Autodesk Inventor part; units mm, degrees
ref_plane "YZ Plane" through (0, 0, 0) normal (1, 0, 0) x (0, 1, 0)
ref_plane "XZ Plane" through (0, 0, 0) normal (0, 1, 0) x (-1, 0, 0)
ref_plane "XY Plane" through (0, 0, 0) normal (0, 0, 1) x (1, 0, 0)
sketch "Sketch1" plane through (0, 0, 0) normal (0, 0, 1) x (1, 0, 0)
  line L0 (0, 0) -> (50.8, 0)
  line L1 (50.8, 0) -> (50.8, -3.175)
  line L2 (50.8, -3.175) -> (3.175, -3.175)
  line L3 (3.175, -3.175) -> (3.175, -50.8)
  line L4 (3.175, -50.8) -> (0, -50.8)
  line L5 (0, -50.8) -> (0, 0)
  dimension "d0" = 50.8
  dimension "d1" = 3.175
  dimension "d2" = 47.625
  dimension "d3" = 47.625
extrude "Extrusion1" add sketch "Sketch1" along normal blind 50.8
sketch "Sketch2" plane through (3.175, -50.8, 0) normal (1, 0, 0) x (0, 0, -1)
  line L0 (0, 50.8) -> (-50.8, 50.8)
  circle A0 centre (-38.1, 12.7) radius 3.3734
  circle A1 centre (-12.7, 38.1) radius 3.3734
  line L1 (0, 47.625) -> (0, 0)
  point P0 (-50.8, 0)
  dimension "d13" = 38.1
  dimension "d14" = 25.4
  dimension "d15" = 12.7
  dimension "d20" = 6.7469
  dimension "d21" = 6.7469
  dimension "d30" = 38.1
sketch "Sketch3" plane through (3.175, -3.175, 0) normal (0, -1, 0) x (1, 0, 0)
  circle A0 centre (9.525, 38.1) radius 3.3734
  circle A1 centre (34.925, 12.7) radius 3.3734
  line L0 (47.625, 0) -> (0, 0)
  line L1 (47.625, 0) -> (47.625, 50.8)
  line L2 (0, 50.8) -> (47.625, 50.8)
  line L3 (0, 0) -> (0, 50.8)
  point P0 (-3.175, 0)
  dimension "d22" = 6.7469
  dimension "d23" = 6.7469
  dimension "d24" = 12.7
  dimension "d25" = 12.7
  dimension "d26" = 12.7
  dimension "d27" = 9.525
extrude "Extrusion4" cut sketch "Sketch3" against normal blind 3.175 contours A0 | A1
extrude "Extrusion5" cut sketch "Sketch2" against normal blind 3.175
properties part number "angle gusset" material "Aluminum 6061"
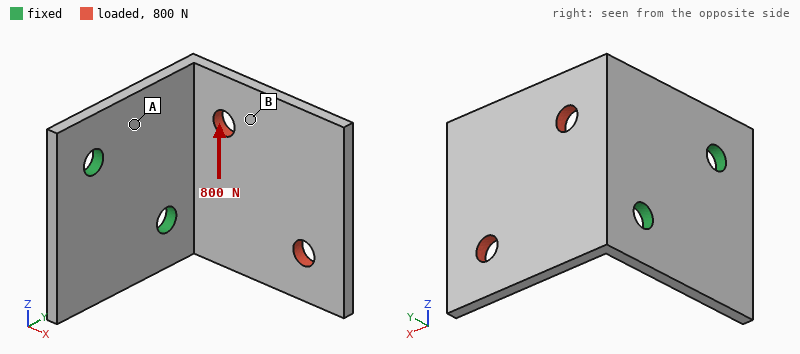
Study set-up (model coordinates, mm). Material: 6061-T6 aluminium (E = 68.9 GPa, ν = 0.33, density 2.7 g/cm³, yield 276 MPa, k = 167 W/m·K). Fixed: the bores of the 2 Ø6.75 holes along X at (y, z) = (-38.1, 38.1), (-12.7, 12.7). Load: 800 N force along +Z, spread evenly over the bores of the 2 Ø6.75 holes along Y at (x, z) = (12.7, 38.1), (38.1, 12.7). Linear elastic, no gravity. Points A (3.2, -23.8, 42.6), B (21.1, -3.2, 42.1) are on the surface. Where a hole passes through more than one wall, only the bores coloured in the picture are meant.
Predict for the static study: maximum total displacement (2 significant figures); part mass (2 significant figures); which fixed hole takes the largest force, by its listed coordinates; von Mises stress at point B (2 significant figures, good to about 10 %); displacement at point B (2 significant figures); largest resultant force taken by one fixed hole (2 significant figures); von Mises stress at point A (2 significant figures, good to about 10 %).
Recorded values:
0.80 mm
42 g
(-12.7, 12.7)
23 MPa
0.42 mm
860 N
63 MPa
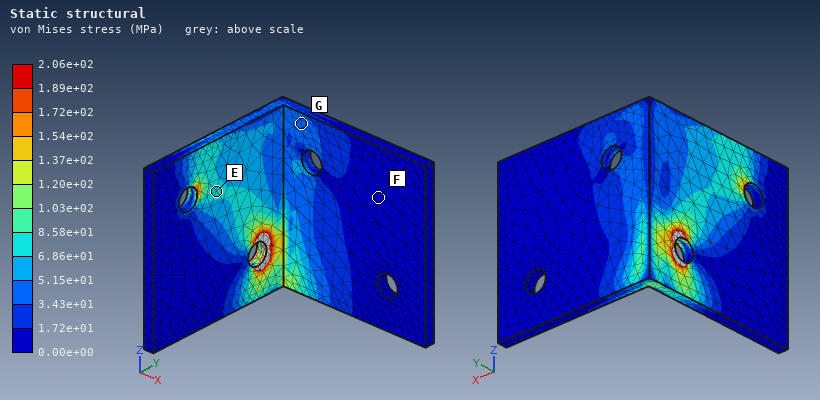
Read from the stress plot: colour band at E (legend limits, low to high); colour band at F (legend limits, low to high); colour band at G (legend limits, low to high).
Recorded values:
6.86e+01 to 8.58e+01 MPa
0.00e+00 to 1.72e+01 MPa
3.43e+01 to 5.15e+01 MPa
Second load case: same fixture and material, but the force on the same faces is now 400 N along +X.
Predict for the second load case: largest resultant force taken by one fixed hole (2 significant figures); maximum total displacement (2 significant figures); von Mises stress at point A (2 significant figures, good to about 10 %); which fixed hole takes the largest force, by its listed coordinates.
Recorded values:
380 N
0.29 mm
22 MPa
(-12.7, 12.7)
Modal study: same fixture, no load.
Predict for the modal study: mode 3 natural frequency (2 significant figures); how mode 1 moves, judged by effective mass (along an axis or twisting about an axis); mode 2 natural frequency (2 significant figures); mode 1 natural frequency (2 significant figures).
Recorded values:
2300 Hz
along Y
1300 Hz
770 Hz
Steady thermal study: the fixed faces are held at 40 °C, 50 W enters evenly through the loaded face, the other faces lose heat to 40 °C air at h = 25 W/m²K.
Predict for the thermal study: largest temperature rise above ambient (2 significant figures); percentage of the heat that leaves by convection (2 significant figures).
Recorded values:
78 K
17 %
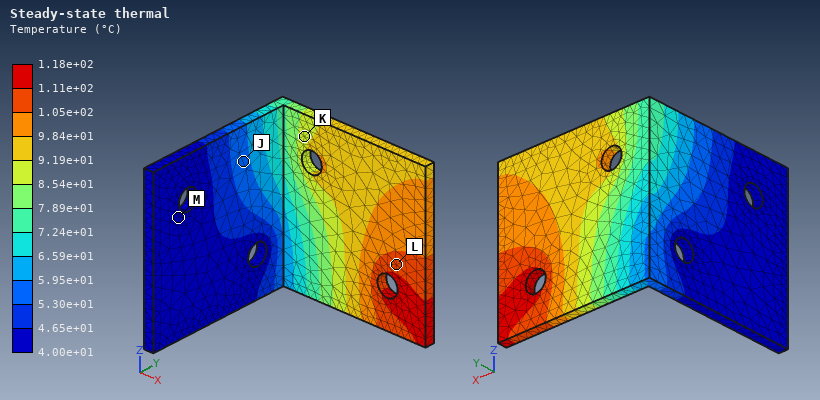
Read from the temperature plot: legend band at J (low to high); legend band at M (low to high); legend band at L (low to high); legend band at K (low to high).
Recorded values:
5.30e+01 to 5.95e+01 °C
4.00e+01 to 4.65e+01 °C
1.05e+02 to 1.11e+02 °C
8.54e+01 to 9.19e+01 °C
